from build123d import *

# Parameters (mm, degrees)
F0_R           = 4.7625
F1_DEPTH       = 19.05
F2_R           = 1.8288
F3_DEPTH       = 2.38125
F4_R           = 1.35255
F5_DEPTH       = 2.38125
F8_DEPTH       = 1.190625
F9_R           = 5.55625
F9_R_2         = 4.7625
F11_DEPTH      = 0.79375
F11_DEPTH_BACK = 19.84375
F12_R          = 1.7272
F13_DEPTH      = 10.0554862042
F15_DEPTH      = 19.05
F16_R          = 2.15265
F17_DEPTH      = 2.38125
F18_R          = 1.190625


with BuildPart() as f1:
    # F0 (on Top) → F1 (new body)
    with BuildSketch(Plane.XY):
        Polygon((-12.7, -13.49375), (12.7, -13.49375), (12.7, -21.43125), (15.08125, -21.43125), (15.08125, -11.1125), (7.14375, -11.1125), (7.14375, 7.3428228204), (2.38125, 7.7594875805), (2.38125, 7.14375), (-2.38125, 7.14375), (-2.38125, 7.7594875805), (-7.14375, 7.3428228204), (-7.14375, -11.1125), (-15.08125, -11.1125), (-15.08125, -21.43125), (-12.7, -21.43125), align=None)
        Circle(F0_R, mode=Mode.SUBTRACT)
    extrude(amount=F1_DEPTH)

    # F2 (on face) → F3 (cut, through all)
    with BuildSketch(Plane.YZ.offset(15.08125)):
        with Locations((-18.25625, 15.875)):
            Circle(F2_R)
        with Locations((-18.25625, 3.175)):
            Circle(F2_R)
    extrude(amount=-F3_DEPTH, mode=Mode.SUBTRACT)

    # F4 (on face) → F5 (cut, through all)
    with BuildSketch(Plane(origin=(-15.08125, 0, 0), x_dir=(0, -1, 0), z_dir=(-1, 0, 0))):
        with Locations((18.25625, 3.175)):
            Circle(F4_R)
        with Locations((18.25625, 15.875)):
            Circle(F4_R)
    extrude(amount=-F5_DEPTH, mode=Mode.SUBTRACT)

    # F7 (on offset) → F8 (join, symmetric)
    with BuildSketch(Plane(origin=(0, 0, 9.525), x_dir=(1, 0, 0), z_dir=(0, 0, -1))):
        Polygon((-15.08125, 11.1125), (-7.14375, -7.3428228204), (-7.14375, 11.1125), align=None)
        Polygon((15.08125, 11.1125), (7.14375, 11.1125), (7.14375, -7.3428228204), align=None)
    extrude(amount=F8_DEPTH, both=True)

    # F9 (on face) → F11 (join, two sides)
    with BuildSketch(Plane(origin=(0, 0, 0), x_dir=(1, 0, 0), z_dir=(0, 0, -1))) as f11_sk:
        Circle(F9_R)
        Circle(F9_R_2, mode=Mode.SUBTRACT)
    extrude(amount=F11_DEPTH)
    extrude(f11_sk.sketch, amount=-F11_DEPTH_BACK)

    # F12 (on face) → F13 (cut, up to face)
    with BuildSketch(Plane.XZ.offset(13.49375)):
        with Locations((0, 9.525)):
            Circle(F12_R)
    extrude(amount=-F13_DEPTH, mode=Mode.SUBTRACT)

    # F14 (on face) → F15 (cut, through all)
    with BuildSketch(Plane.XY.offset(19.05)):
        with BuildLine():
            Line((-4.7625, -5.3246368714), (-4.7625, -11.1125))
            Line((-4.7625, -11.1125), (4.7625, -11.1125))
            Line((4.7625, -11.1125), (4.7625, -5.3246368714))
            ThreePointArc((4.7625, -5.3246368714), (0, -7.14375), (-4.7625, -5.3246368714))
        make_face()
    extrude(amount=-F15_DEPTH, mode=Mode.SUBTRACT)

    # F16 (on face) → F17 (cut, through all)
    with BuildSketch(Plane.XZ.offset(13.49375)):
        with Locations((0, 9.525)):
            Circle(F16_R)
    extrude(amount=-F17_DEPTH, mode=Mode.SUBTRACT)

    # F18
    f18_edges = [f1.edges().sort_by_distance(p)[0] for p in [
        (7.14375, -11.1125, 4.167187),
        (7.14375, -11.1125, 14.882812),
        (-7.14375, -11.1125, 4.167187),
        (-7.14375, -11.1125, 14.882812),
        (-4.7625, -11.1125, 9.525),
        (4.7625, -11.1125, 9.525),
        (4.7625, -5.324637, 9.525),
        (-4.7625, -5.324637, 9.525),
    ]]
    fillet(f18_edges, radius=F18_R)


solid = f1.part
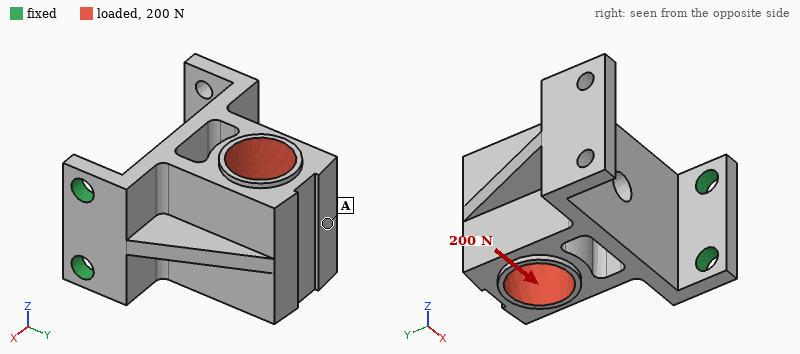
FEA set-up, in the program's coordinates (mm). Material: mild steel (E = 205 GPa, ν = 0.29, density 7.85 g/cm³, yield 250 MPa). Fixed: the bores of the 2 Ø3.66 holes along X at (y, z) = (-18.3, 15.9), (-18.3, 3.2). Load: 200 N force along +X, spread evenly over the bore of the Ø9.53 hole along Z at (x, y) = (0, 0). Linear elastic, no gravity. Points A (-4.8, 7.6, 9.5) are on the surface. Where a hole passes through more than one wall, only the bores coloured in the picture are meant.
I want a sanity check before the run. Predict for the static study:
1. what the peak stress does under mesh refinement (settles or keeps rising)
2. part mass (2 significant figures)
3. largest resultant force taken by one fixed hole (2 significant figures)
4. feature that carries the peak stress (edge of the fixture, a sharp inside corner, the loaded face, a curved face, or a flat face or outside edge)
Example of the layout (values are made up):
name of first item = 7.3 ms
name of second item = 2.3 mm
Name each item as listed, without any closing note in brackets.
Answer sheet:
what the peak stress does under mesh refinement = keeps rising
part mass = 41 g
largest resultant force taken by one fixed hole = 110 N
feature that carries the peak stress = edge of the fixture
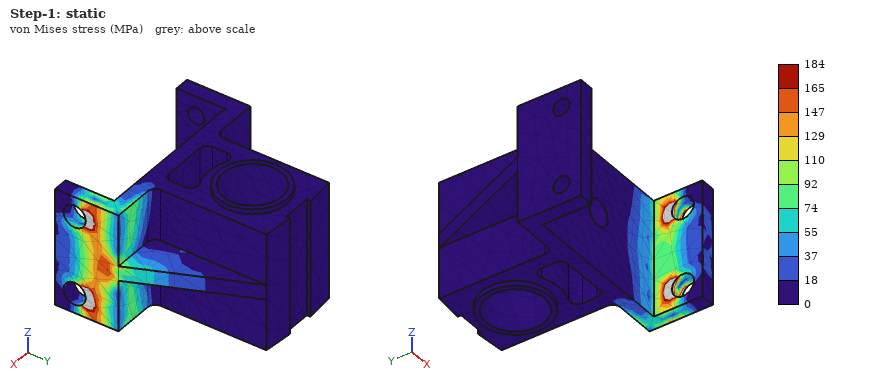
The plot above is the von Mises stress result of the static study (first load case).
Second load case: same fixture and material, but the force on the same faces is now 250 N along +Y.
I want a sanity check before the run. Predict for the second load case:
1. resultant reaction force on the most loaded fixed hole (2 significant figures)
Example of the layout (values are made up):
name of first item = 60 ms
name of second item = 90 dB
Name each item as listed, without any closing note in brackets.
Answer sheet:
resultant reaction force on the most loaded fixed hole = 130 N
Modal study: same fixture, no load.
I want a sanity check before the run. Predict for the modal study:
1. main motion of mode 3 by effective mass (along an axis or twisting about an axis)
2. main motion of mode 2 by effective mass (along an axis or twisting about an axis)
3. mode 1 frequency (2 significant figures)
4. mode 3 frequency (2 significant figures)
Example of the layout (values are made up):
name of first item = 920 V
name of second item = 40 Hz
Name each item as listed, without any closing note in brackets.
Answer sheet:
main motion of mode 3 by effective mass = twisting about X
main motion of mode 2 by effective mass = along Z
mode 1 frequency = 1000 Hz
mode 3 frequency = 4000 Hz
